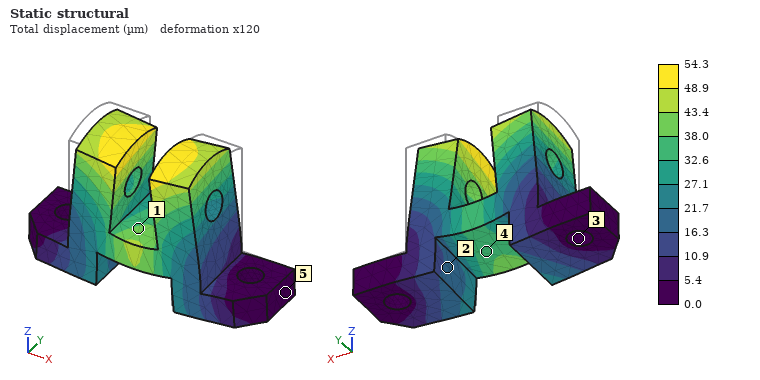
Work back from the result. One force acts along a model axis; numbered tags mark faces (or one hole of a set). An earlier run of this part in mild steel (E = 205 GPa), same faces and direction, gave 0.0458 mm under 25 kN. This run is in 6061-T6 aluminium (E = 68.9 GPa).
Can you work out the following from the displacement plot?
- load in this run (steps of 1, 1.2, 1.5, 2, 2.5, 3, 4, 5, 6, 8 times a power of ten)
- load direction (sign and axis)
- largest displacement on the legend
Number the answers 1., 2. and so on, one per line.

1. 10 kN
2. -Z
3. 54.3 µm
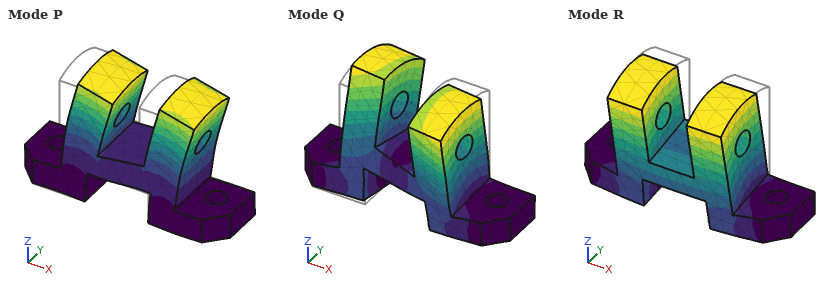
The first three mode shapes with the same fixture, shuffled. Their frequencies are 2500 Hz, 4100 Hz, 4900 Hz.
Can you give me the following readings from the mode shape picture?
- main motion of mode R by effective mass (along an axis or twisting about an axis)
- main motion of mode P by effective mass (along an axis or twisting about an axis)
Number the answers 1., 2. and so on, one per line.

1. along Y
2. along X
